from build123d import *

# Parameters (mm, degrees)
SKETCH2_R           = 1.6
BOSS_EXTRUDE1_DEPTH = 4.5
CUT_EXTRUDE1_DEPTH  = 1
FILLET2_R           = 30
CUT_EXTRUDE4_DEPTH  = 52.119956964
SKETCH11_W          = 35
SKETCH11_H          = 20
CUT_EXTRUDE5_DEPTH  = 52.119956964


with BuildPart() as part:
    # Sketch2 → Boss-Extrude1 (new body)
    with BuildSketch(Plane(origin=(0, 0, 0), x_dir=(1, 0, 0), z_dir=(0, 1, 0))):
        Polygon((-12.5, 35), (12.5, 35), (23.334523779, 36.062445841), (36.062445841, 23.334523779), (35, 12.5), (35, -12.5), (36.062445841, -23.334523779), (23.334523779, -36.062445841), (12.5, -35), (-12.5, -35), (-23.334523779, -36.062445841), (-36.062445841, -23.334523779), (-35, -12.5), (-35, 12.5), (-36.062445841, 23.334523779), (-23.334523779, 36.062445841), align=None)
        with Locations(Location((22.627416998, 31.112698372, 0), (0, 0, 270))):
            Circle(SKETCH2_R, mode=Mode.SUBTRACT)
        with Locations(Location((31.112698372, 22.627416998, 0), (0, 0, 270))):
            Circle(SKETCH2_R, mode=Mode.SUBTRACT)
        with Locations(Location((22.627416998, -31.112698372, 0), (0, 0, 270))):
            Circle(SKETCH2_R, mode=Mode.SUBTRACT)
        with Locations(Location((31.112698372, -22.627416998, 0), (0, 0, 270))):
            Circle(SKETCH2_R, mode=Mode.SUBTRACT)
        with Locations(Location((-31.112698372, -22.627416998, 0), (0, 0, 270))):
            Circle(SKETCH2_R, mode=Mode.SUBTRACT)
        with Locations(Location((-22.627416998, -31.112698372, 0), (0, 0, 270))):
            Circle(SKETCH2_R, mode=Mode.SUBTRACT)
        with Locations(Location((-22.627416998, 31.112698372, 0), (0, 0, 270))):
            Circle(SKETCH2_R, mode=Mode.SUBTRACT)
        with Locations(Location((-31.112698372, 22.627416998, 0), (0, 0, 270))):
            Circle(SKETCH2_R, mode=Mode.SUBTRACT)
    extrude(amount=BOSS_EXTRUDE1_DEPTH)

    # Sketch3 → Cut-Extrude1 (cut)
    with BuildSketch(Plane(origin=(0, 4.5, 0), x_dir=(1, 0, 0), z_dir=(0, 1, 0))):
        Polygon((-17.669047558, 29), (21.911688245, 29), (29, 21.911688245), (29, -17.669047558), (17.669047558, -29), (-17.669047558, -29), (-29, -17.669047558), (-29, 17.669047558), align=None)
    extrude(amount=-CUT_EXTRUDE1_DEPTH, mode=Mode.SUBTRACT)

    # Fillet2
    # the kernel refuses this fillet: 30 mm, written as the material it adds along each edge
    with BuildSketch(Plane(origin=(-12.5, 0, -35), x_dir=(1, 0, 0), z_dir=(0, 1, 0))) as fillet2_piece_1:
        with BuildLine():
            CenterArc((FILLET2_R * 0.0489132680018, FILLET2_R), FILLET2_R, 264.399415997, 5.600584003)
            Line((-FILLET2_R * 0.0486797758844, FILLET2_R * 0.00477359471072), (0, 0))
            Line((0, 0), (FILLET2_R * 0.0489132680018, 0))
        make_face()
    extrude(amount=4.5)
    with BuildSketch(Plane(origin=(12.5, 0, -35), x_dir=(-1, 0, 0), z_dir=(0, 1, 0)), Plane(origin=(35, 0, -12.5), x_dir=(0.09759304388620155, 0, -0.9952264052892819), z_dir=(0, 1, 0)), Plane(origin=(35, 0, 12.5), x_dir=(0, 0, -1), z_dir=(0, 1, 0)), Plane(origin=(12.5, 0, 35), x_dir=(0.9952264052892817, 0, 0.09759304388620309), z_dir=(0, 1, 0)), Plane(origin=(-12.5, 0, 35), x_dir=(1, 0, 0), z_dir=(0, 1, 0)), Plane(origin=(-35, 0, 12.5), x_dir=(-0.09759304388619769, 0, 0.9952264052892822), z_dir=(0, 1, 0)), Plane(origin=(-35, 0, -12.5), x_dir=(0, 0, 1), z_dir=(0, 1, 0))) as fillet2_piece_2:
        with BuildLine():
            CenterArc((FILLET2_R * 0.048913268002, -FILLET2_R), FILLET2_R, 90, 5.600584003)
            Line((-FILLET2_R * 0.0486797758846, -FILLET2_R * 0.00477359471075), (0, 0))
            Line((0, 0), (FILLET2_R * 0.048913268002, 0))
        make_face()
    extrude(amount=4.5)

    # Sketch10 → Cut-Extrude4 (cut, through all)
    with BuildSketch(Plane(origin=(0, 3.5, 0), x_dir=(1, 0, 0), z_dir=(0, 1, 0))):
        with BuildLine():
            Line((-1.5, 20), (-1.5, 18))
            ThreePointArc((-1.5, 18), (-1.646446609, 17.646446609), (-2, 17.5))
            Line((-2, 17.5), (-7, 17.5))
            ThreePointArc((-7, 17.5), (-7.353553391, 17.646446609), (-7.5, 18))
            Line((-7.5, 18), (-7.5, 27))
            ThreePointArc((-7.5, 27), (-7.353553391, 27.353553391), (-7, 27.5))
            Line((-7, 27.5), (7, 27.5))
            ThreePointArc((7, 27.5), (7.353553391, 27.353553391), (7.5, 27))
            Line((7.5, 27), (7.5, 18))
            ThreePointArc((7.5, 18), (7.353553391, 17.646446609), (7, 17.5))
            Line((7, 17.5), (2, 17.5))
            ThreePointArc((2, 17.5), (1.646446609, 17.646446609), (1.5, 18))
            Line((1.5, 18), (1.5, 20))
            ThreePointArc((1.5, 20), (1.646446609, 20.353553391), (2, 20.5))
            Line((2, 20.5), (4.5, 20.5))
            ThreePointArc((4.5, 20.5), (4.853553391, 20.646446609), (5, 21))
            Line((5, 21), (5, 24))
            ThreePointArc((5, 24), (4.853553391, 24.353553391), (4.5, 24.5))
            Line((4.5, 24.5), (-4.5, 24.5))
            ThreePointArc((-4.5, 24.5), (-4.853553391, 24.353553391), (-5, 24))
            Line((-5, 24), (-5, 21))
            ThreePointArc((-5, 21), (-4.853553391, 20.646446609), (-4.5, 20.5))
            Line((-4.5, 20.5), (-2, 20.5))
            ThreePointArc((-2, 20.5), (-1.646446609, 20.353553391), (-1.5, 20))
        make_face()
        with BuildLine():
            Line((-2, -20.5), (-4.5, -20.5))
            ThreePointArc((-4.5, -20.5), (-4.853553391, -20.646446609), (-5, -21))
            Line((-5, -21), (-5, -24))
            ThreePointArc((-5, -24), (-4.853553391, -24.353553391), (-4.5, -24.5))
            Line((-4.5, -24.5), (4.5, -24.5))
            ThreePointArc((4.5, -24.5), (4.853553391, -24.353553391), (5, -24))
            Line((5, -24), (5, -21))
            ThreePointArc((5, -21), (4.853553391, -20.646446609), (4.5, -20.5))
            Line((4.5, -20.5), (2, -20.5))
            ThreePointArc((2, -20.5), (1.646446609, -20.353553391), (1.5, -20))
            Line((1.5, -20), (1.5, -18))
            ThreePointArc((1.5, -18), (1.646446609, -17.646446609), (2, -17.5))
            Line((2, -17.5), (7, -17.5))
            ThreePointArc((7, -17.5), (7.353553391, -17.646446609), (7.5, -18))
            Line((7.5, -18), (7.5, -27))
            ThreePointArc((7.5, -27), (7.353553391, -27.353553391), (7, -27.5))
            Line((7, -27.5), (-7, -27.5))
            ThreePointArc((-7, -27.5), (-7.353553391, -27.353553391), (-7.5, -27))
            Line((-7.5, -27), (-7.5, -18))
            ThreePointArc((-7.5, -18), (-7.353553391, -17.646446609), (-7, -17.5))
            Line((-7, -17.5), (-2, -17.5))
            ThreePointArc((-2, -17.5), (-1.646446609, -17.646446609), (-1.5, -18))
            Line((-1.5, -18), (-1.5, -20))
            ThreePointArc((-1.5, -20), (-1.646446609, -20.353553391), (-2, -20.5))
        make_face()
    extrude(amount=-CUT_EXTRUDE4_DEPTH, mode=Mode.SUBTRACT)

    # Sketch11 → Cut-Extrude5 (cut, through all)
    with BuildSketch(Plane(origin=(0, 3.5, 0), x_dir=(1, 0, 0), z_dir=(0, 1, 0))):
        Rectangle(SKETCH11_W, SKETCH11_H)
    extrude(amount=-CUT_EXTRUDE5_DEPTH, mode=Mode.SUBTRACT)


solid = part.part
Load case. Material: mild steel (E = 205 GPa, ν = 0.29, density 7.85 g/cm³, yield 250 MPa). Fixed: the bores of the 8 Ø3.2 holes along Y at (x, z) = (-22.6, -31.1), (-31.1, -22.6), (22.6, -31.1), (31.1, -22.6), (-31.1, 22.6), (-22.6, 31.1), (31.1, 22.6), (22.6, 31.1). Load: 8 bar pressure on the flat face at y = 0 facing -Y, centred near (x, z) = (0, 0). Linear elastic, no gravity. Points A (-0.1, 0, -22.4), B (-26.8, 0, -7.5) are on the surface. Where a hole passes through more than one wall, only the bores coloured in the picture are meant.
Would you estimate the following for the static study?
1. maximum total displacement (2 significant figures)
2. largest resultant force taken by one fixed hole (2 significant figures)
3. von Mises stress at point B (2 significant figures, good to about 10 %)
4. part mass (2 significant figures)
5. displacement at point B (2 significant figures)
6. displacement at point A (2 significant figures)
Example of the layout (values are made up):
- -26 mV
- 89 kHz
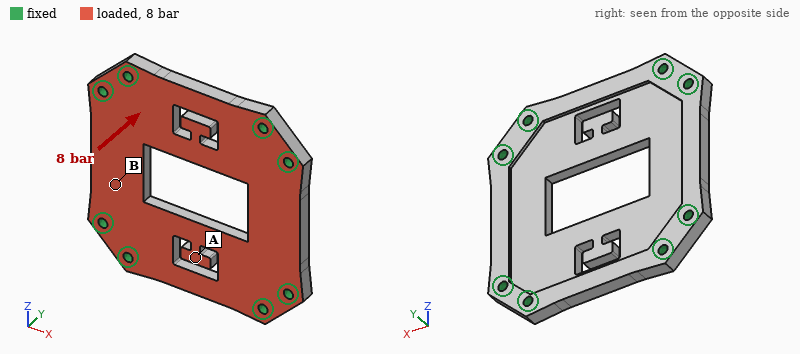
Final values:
- 34 µm
- 400 N
- 28 MPa
- 120 g
- 11 µm
- 25 µm
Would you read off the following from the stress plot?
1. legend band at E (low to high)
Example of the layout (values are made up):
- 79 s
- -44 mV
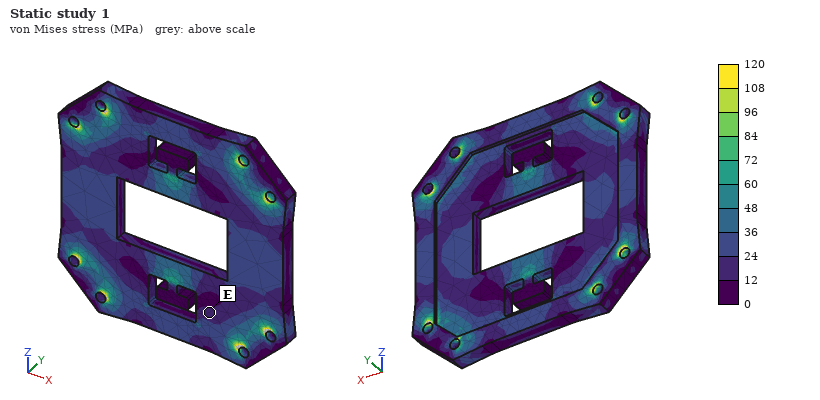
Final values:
- 12 to 24 MPa
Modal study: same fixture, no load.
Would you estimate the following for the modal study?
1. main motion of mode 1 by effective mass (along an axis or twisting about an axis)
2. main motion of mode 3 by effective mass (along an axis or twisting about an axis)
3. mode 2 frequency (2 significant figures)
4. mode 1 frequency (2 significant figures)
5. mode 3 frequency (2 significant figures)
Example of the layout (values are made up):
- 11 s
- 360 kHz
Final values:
- along Y
- twisting about Z
- 7600 Hz
- 6300 Hz
- 9600 Hz
